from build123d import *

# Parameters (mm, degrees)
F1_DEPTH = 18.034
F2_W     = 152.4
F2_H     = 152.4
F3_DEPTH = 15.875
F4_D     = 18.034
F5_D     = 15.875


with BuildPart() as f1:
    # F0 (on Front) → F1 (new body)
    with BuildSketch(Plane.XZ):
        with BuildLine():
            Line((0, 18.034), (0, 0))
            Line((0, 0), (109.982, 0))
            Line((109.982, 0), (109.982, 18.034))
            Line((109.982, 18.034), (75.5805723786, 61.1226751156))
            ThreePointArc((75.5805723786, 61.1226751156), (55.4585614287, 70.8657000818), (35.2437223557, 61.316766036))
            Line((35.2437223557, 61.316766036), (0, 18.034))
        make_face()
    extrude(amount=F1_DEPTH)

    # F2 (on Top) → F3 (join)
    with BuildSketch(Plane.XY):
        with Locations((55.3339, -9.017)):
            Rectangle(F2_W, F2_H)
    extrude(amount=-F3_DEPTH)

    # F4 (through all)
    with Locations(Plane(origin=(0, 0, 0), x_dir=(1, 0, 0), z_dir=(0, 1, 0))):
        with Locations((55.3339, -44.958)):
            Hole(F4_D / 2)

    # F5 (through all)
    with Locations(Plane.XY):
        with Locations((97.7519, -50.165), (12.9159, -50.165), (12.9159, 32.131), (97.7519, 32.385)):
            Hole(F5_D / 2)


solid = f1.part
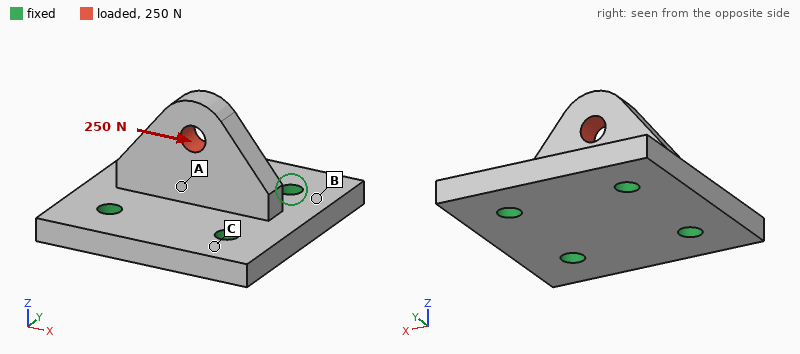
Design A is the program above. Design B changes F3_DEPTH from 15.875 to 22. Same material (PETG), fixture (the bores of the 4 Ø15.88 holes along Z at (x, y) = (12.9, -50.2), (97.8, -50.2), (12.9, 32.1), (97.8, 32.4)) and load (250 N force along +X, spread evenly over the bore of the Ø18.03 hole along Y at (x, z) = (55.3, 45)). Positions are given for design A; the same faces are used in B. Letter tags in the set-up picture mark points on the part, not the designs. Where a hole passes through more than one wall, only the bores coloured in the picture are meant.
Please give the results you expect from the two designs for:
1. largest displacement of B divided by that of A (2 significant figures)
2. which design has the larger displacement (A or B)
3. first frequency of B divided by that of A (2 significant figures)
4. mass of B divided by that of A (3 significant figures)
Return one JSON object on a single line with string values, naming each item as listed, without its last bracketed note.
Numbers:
{"largest displacement of B divided by that of A": "0.78", "which design has the larger displacement": "A", "first frequency of B divided by that of A": "1.1", "mass of B divided by that of A": "1.30"}
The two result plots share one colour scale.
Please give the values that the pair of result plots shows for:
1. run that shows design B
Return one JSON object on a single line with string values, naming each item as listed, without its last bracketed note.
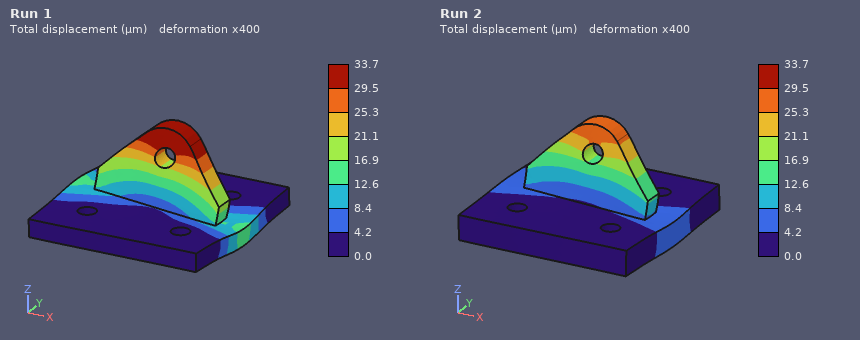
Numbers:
{"run that shows design B": "Run 2"}
